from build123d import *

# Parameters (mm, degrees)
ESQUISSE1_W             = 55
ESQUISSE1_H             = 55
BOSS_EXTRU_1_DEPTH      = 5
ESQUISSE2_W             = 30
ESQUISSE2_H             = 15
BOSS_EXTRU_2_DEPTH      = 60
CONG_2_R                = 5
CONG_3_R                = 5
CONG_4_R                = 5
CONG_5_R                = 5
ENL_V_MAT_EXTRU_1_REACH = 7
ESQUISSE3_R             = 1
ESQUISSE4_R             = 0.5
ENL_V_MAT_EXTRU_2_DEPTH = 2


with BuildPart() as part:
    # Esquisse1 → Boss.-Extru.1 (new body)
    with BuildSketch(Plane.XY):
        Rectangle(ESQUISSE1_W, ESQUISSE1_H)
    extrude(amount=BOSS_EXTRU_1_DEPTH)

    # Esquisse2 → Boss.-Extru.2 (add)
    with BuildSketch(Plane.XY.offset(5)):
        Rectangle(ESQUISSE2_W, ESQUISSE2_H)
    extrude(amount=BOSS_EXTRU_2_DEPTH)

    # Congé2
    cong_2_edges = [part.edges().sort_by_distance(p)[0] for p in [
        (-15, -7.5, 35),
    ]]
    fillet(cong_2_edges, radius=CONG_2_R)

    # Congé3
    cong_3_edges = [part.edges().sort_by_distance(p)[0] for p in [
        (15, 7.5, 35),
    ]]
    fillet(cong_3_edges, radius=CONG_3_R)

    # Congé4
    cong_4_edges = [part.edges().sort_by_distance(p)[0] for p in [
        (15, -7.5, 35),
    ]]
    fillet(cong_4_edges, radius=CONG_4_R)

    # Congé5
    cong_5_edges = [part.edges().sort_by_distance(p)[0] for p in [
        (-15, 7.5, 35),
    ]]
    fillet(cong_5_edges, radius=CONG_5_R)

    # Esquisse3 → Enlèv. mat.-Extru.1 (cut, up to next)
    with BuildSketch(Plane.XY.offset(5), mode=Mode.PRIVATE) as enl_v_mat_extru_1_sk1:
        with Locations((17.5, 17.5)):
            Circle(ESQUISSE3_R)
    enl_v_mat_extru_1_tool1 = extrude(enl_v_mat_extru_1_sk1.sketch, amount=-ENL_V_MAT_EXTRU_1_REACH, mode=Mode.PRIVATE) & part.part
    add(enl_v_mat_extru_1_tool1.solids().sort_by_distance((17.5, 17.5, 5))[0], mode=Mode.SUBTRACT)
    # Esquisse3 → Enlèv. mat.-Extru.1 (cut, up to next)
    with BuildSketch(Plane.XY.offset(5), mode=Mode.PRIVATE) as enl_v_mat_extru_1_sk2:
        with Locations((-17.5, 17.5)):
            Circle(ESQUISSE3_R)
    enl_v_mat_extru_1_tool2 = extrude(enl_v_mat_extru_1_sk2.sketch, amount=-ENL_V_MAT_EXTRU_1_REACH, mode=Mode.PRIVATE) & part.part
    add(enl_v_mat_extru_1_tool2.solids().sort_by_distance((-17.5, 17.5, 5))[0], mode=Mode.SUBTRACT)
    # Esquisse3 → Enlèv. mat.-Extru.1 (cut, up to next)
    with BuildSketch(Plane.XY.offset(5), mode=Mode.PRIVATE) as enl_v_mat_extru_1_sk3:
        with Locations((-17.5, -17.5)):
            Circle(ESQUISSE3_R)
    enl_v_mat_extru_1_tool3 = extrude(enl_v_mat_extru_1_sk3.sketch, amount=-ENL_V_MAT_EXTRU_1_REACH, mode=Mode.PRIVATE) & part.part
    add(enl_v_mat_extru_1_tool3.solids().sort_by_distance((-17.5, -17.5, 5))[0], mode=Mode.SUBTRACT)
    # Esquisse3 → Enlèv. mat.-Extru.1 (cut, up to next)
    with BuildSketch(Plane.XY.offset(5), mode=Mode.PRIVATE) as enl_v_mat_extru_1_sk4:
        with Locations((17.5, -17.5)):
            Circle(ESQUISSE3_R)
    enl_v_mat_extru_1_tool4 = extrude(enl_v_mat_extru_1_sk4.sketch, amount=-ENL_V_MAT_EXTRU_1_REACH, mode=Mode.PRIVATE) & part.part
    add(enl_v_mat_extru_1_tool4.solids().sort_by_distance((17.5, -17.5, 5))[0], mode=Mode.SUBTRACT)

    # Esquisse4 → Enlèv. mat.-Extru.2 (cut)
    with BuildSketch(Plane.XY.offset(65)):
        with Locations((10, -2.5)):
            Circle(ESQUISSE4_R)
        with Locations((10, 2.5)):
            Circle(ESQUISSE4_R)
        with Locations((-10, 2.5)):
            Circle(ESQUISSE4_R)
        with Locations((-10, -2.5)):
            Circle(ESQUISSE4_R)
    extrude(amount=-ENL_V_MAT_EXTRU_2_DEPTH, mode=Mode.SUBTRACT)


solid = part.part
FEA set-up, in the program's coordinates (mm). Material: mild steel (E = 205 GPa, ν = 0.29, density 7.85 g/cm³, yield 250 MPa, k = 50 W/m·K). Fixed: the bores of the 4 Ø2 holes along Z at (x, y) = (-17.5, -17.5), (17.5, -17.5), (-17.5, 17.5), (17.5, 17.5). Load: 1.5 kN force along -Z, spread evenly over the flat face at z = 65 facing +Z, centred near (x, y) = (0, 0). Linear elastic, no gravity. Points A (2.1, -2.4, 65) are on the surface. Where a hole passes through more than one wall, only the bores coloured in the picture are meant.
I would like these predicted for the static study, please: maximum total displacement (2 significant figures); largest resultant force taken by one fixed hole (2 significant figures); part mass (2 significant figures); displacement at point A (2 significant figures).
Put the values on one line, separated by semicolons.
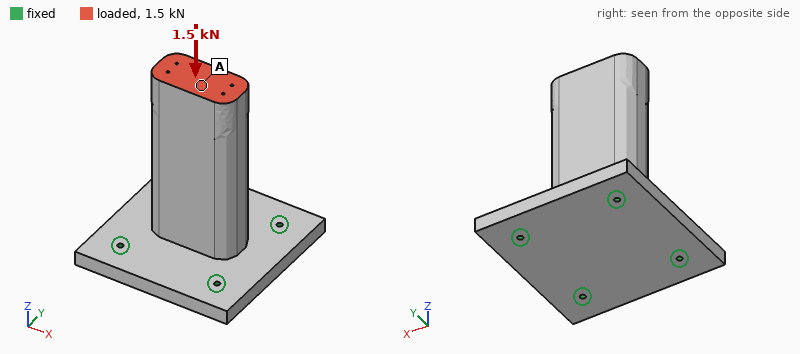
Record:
5.3 µm; 390 N; 320 g; 5.3 µm
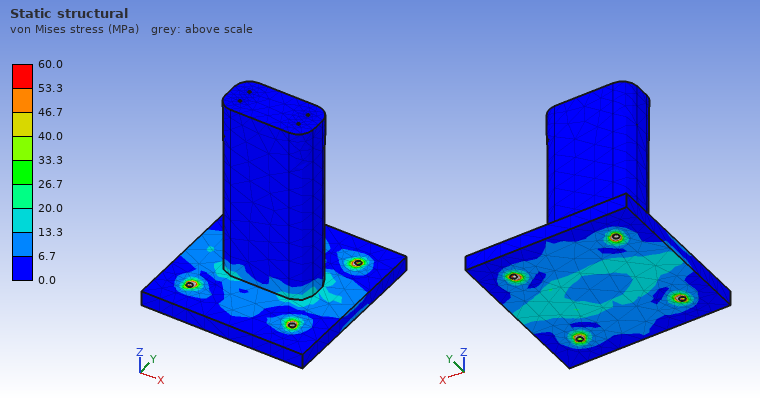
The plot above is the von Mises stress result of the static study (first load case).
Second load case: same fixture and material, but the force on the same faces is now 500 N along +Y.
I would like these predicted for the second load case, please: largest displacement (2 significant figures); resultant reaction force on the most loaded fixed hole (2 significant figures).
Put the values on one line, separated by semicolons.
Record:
55 µm; 530 N
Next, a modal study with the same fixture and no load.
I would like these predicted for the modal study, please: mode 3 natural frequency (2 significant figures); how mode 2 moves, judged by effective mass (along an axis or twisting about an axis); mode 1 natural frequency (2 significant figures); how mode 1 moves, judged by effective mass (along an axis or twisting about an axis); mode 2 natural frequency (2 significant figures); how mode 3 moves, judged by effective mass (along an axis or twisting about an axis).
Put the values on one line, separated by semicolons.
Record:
5900 Hz; along X; 1900 Hz; along Y; 2600 Hz; along Z
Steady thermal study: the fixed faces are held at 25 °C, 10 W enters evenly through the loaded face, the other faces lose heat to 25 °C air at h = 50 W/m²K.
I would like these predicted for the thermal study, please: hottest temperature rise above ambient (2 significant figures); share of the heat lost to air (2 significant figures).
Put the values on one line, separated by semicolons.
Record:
27 K; 45 %
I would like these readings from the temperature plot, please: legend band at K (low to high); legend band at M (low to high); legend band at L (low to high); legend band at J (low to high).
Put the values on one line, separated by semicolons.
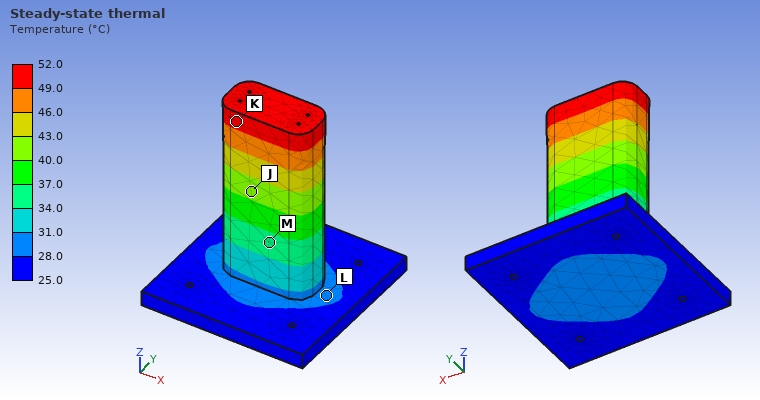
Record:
49.0 to 52.0 °C; 34.0 to 37.0 °C; 28.0 to 31.0 °C; 40.0 to 43.0 °C
